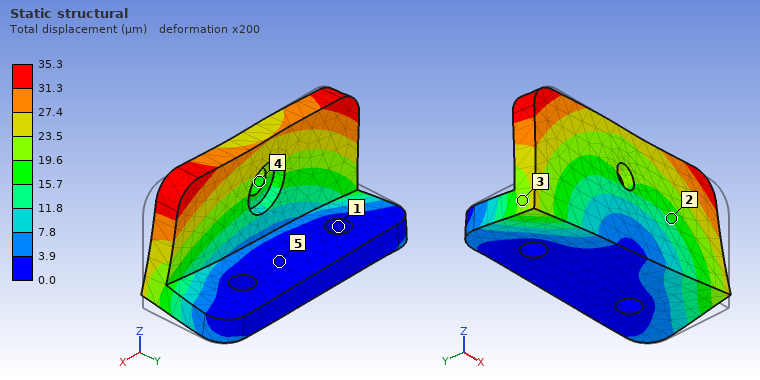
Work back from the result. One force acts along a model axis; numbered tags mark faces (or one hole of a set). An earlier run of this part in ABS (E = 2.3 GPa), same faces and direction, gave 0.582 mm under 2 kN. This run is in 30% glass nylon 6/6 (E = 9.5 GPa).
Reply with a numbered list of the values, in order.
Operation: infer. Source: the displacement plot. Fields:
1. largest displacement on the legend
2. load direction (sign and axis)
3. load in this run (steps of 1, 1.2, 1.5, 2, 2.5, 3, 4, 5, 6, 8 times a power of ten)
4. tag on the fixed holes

1. 35.3 µm
2. -X
3. 500 N
4. 1
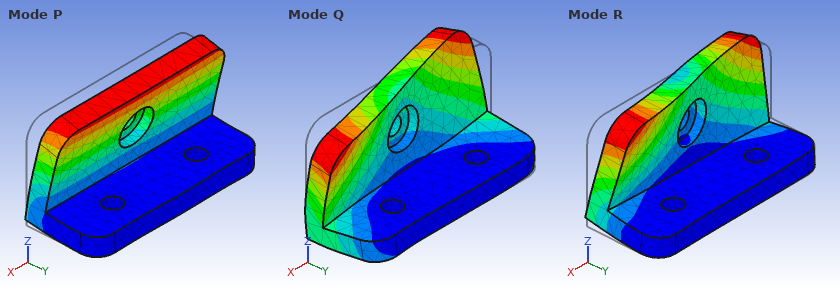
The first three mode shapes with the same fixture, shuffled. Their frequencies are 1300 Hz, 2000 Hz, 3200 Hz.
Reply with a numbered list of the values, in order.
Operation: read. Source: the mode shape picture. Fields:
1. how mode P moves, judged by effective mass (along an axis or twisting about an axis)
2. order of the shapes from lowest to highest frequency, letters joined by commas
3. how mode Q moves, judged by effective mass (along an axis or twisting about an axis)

1. along Y
2. P, R, Q
3. along X
